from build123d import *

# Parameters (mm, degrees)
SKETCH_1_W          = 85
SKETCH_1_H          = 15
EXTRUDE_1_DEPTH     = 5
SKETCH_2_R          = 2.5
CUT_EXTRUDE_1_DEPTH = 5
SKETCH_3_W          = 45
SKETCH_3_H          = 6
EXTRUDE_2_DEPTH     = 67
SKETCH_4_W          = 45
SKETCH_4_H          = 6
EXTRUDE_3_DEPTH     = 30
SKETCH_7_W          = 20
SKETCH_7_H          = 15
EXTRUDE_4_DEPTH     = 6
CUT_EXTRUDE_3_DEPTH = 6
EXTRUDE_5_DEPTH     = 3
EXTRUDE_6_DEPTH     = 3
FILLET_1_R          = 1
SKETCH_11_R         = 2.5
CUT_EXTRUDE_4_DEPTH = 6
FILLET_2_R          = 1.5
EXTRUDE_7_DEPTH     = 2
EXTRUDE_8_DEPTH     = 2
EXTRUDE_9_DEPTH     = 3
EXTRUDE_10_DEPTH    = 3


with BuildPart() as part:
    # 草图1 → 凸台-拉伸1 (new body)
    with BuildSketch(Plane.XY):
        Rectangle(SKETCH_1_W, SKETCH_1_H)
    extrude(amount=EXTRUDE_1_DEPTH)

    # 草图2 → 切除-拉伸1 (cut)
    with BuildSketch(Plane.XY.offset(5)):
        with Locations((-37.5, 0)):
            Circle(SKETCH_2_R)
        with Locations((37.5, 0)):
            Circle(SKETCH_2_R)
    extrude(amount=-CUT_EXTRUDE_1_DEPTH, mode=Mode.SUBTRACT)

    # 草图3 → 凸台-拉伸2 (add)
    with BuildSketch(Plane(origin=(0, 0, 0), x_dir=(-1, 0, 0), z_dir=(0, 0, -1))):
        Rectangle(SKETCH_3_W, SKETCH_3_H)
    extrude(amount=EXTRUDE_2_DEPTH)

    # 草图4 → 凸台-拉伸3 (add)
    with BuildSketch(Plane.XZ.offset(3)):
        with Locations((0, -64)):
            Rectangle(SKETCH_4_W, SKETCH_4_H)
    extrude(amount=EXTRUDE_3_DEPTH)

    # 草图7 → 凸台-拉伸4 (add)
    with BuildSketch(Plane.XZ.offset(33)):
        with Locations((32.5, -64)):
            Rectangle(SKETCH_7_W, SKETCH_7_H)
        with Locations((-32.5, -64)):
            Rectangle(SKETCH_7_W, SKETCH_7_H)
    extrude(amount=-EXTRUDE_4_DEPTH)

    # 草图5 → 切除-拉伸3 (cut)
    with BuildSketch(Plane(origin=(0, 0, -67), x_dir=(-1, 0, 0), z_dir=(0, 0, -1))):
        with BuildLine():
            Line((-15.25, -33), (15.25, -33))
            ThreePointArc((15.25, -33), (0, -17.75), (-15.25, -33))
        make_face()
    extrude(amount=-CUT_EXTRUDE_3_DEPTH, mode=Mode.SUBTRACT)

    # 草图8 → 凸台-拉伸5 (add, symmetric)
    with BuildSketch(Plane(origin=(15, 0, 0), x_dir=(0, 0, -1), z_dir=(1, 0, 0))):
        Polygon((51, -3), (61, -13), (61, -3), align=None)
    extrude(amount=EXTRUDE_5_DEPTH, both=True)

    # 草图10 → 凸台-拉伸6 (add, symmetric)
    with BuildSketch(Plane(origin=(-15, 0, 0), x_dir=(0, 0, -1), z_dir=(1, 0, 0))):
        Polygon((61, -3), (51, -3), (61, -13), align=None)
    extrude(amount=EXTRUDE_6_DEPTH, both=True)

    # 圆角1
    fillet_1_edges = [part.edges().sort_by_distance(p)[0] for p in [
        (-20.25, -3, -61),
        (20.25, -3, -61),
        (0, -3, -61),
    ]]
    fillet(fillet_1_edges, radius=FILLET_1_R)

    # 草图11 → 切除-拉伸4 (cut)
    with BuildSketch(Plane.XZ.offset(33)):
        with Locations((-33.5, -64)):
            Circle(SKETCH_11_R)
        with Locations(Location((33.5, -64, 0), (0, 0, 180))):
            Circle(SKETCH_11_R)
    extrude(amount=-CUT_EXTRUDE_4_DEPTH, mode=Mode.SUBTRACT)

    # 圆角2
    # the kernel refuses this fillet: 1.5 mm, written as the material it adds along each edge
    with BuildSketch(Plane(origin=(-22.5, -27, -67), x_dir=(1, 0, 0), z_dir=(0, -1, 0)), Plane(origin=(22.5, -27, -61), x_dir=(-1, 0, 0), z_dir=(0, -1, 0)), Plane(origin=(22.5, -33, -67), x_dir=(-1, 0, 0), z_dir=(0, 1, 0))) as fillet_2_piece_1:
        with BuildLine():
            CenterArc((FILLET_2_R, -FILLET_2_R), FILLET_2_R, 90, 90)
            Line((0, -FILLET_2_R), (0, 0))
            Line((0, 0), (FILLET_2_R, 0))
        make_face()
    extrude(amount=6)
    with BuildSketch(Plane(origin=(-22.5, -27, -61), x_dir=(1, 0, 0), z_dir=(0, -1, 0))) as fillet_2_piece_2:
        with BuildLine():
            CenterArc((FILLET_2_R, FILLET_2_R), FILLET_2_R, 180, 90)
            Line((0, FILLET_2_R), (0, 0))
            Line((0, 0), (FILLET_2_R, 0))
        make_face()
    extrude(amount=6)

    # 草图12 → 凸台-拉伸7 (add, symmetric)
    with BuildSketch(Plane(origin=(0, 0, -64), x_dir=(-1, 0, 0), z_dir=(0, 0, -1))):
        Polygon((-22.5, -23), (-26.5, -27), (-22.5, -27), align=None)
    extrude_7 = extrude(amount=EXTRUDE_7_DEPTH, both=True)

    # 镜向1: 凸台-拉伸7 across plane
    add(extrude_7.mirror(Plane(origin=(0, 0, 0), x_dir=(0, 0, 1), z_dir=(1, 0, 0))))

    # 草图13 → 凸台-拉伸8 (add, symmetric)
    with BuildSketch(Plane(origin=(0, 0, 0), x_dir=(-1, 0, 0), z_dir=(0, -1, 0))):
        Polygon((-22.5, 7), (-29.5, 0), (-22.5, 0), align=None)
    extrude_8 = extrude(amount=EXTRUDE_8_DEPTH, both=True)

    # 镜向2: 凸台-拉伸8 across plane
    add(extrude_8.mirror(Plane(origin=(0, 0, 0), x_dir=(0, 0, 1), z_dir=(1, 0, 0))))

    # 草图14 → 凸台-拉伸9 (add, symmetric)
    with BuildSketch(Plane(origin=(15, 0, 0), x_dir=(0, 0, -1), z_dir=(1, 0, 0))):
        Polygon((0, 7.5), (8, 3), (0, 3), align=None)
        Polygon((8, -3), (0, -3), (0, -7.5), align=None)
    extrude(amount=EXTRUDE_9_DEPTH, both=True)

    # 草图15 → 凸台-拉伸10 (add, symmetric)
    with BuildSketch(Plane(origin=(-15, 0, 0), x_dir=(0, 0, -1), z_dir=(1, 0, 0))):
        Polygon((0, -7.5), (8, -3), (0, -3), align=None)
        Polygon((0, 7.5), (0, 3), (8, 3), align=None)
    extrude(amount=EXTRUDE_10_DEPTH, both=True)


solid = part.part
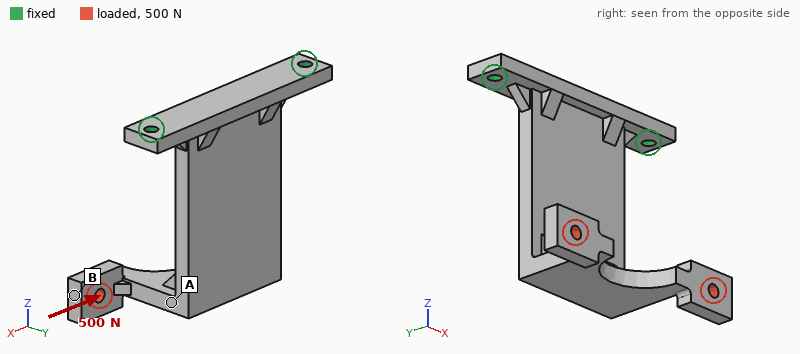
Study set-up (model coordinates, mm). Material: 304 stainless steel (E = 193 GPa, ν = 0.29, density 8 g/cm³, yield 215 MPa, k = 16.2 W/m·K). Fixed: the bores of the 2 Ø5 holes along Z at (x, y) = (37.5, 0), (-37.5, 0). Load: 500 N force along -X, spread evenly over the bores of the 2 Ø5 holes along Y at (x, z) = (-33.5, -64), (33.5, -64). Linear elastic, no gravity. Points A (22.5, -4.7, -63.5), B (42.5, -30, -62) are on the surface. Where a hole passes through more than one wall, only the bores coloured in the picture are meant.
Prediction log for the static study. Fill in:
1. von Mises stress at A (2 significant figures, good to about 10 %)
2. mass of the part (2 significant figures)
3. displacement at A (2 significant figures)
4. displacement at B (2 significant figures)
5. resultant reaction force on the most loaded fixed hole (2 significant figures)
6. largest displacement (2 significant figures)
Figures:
10 MPa
280 g
0.079 mm
0.18 mm
640 N
0.19 mm
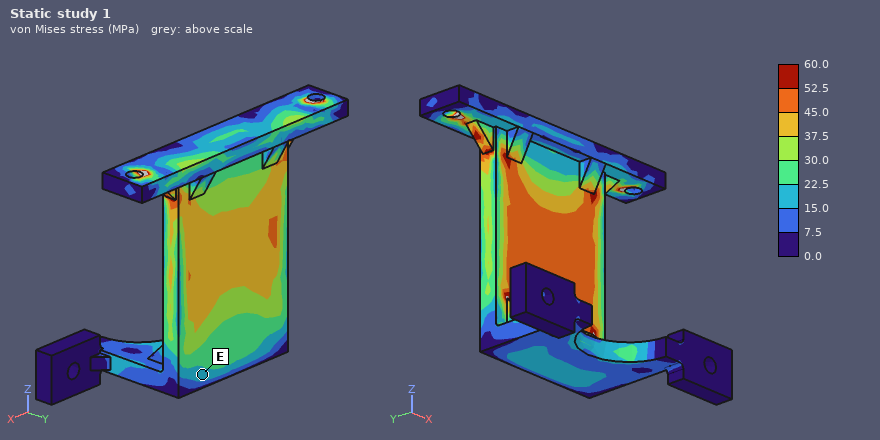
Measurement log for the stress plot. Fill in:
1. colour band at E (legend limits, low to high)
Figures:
15.0 to 22.5 MPa
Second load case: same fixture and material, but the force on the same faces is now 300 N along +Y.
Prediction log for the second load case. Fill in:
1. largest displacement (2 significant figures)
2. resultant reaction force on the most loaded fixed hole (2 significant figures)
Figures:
0.53 mm
150 N
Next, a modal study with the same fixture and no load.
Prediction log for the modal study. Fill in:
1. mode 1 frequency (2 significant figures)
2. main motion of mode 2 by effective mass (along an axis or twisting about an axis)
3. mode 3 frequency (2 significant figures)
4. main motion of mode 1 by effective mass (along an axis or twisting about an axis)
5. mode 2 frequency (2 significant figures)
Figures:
370 Hz
along X
1800 Hz
along Y
1100 Hz
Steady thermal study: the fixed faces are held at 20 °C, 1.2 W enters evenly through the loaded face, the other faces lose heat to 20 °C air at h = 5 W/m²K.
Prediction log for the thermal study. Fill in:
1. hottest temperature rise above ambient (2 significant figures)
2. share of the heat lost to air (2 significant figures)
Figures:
27 K
61 %
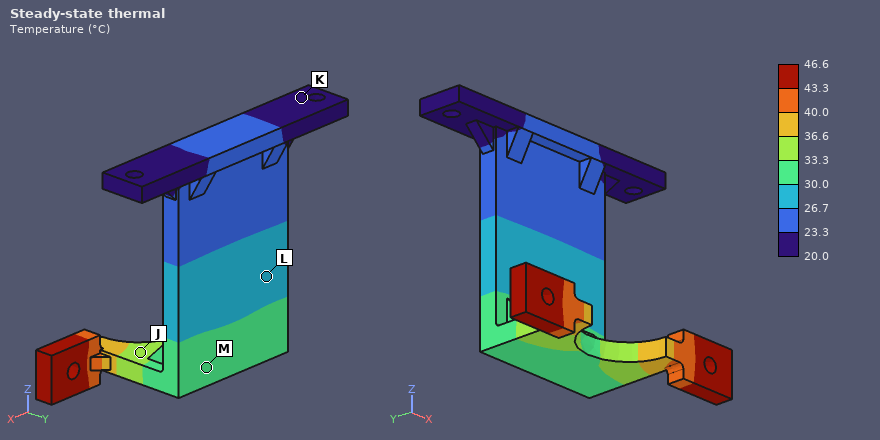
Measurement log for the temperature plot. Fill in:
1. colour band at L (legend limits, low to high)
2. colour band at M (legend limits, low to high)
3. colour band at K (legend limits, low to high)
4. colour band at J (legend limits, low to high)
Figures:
26.7 to 30.0 °C
30.0 to 33.3 °C
20.0 to 23.3 °C
33.3 to 36.6 °C
